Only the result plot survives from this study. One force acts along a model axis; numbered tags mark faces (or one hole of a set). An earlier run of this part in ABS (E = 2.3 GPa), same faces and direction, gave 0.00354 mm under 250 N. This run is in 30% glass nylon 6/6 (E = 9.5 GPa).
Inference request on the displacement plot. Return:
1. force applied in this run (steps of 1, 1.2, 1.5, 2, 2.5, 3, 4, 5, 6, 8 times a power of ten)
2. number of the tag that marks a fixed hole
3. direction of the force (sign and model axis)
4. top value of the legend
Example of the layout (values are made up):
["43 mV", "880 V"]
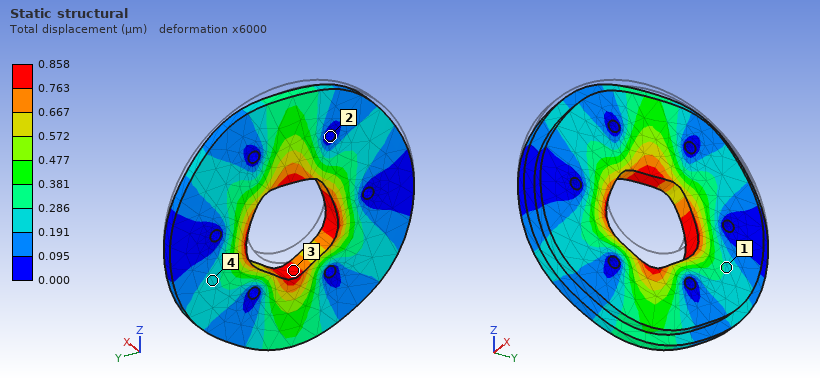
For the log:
["250 N", "2", "-Z", "0.858 µm"]
